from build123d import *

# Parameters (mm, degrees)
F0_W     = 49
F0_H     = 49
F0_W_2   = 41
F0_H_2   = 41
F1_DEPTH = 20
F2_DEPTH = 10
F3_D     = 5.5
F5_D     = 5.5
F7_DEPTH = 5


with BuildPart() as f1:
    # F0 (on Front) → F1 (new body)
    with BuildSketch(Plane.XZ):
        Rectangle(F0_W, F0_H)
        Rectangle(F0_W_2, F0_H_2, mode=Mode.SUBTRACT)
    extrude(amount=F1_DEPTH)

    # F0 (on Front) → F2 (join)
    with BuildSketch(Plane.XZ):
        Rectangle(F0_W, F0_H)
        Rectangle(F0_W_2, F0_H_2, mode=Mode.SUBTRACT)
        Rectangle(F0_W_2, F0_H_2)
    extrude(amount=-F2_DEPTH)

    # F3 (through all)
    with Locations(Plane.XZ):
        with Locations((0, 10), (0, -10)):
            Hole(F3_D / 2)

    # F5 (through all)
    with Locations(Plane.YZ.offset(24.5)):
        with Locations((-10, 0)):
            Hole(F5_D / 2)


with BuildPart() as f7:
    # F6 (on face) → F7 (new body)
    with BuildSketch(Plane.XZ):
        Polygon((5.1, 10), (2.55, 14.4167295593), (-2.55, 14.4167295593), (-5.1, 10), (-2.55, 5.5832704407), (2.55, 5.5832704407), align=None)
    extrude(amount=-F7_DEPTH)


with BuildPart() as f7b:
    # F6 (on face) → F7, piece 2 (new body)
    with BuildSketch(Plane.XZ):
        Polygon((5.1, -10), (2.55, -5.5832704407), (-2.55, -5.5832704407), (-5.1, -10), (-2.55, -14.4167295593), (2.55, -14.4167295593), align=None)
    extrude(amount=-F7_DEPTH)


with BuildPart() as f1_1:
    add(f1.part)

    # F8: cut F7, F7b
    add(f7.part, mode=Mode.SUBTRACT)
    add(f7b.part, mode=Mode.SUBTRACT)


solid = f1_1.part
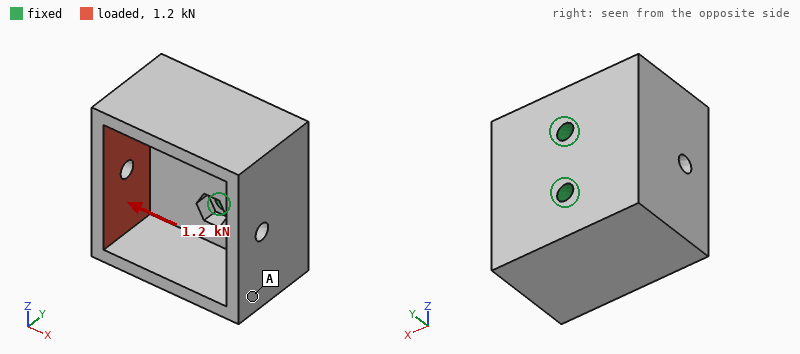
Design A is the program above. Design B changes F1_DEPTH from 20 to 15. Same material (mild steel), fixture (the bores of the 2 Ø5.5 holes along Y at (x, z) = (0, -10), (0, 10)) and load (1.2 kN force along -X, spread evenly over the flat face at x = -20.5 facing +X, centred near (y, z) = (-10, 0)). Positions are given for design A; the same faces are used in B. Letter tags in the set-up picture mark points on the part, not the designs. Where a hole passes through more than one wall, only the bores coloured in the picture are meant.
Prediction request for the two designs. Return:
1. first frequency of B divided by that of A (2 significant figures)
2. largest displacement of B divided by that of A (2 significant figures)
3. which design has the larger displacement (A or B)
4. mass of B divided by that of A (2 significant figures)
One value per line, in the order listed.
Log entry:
1.2
0.78
A
0.90
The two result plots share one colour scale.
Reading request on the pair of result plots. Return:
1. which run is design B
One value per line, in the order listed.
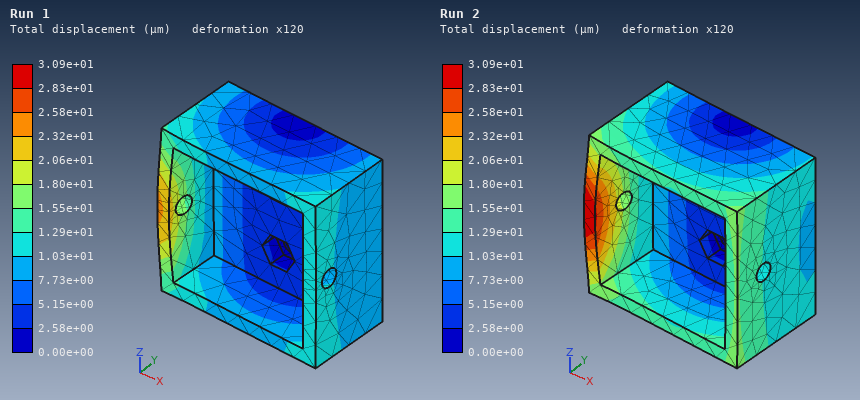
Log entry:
Run 1
